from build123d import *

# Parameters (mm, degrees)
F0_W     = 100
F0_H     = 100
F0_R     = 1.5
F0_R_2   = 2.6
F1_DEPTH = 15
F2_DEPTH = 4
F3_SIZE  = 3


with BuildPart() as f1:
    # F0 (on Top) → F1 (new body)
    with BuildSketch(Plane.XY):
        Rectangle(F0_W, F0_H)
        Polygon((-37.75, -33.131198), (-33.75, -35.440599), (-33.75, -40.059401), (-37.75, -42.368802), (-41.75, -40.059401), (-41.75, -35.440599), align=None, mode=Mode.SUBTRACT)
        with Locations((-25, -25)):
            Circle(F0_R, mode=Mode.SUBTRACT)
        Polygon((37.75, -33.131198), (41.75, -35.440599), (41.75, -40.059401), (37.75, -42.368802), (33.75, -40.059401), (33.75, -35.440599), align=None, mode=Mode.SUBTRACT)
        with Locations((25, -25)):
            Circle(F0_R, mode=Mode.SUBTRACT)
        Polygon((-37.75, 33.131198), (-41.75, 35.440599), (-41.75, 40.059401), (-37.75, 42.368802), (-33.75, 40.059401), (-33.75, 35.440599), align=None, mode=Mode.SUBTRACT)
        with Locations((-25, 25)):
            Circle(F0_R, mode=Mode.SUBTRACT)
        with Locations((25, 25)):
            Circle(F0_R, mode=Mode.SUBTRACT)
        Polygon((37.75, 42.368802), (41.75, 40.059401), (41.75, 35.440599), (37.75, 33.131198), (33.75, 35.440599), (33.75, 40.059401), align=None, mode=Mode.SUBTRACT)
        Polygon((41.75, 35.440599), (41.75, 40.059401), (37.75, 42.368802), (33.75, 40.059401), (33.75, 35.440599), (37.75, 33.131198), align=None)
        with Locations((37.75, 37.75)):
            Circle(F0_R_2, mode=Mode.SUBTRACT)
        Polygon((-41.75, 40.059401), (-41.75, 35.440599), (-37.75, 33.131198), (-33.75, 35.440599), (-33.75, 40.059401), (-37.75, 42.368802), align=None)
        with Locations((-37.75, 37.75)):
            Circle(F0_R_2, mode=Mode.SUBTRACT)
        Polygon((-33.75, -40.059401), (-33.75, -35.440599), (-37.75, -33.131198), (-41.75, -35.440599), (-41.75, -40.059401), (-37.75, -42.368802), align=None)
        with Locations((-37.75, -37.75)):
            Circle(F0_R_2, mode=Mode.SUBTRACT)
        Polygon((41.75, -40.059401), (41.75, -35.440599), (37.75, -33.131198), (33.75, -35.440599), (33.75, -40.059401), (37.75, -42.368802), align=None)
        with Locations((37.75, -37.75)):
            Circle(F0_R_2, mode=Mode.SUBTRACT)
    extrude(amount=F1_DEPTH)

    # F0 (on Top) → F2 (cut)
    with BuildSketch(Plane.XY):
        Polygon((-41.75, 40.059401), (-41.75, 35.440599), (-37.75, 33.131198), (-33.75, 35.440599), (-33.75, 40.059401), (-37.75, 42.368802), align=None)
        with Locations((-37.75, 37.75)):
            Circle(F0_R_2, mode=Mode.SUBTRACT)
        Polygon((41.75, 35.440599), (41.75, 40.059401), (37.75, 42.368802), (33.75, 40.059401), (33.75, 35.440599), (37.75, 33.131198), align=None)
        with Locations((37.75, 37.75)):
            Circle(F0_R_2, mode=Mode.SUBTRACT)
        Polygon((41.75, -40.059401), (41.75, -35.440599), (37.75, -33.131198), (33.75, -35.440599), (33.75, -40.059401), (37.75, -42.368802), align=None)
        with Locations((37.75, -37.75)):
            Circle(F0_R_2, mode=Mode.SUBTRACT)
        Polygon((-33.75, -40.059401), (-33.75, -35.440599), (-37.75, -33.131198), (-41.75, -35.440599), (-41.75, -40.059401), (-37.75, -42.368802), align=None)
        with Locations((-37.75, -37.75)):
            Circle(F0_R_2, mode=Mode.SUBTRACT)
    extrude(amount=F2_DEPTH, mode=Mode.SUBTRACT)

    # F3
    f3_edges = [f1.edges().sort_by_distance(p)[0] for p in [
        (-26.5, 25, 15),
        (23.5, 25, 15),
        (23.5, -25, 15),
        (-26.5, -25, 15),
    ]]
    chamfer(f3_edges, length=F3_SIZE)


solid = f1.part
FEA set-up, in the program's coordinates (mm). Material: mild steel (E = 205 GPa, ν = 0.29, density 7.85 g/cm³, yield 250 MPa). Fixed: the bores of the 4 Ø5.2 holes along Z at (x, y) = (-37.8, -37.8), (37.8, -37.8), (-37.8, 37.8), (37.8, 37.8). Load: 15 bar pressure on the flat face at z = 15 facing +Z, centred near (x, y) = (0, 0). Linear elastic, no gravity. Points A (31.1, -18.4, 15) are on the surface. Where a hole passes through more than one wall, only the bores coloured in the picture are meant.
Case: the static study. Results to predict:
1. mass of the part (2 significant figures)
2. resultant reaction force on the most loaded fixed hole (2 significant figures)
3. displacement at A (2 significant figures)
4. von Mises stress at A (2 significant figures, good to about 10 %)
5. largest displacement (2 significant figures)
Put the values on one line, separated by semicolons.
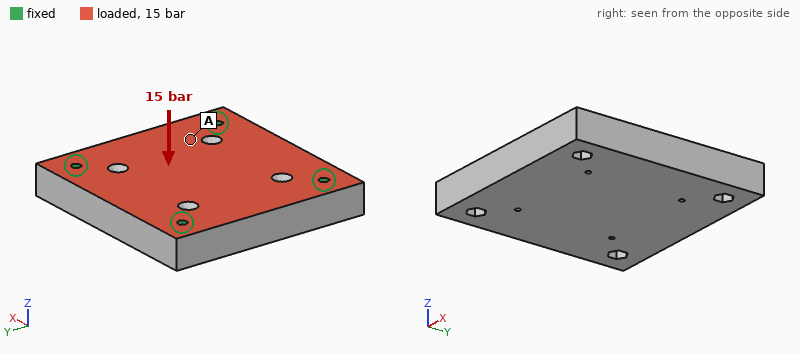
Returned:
1.2 kg; 3.7 kN; 5.7 µm; 7.4 MPa; 10.0 µm
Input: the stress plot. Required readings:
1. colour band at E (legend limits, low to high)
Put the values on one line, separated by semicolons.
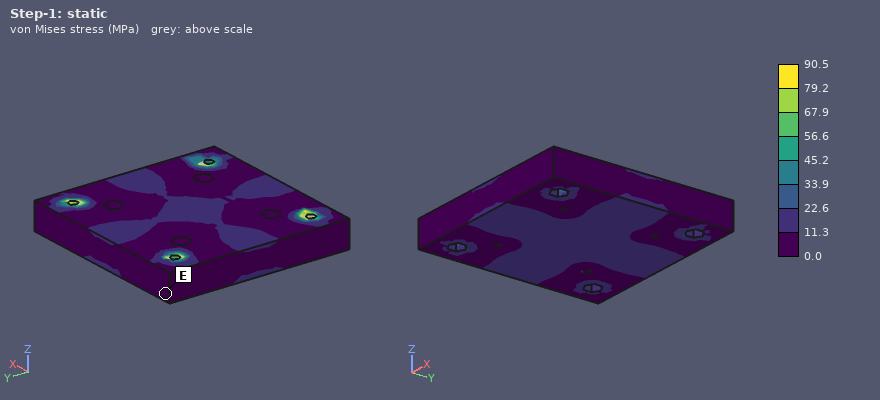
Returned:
0.0 to 11.3 MPa
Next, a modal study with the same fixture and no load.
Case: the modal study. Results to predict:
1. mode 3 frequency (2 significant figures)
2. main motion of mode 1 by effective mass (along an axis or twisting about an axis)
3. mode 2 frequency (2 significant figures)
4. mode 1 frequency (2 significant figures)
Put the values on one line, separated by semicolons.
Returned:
10 kHz; along Z; 10 kHz; 6600 Hz
